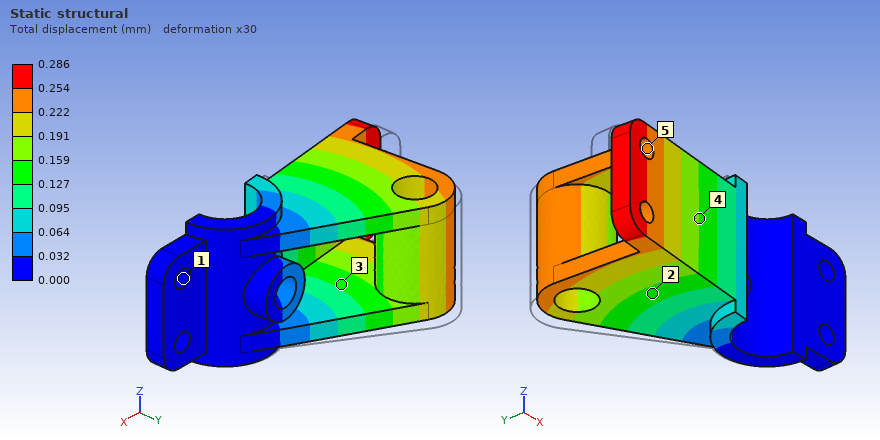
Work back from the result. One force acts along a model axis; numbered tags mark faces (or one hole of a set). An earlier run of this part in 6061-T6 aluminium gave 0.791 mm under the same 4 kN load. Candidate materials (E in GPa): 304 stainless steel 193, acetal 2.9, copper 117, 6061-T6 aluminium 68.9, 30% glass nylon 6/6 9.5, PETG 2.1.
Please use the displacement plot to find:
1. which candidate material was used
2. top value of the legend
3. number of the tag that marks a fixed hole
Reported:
304 stainless steel
0.286 mm
1
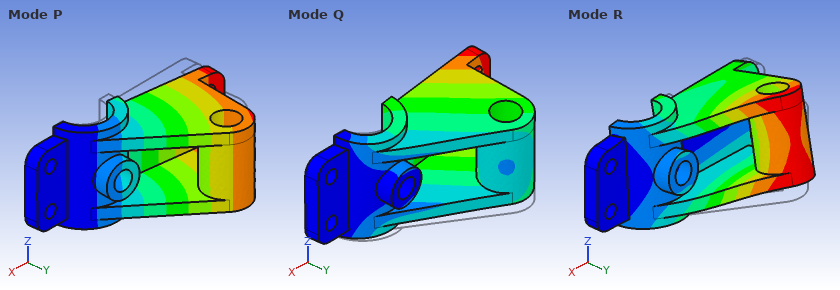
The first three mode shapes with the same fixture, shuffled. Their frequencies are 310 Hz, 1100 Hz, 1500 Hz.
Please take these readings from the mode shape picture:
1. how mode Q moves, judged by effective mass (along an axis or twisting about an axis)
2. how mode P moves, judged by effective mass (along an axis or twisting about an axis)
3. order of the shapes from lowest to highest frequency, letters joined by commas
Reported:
along Z
along Y
P, Q, R
